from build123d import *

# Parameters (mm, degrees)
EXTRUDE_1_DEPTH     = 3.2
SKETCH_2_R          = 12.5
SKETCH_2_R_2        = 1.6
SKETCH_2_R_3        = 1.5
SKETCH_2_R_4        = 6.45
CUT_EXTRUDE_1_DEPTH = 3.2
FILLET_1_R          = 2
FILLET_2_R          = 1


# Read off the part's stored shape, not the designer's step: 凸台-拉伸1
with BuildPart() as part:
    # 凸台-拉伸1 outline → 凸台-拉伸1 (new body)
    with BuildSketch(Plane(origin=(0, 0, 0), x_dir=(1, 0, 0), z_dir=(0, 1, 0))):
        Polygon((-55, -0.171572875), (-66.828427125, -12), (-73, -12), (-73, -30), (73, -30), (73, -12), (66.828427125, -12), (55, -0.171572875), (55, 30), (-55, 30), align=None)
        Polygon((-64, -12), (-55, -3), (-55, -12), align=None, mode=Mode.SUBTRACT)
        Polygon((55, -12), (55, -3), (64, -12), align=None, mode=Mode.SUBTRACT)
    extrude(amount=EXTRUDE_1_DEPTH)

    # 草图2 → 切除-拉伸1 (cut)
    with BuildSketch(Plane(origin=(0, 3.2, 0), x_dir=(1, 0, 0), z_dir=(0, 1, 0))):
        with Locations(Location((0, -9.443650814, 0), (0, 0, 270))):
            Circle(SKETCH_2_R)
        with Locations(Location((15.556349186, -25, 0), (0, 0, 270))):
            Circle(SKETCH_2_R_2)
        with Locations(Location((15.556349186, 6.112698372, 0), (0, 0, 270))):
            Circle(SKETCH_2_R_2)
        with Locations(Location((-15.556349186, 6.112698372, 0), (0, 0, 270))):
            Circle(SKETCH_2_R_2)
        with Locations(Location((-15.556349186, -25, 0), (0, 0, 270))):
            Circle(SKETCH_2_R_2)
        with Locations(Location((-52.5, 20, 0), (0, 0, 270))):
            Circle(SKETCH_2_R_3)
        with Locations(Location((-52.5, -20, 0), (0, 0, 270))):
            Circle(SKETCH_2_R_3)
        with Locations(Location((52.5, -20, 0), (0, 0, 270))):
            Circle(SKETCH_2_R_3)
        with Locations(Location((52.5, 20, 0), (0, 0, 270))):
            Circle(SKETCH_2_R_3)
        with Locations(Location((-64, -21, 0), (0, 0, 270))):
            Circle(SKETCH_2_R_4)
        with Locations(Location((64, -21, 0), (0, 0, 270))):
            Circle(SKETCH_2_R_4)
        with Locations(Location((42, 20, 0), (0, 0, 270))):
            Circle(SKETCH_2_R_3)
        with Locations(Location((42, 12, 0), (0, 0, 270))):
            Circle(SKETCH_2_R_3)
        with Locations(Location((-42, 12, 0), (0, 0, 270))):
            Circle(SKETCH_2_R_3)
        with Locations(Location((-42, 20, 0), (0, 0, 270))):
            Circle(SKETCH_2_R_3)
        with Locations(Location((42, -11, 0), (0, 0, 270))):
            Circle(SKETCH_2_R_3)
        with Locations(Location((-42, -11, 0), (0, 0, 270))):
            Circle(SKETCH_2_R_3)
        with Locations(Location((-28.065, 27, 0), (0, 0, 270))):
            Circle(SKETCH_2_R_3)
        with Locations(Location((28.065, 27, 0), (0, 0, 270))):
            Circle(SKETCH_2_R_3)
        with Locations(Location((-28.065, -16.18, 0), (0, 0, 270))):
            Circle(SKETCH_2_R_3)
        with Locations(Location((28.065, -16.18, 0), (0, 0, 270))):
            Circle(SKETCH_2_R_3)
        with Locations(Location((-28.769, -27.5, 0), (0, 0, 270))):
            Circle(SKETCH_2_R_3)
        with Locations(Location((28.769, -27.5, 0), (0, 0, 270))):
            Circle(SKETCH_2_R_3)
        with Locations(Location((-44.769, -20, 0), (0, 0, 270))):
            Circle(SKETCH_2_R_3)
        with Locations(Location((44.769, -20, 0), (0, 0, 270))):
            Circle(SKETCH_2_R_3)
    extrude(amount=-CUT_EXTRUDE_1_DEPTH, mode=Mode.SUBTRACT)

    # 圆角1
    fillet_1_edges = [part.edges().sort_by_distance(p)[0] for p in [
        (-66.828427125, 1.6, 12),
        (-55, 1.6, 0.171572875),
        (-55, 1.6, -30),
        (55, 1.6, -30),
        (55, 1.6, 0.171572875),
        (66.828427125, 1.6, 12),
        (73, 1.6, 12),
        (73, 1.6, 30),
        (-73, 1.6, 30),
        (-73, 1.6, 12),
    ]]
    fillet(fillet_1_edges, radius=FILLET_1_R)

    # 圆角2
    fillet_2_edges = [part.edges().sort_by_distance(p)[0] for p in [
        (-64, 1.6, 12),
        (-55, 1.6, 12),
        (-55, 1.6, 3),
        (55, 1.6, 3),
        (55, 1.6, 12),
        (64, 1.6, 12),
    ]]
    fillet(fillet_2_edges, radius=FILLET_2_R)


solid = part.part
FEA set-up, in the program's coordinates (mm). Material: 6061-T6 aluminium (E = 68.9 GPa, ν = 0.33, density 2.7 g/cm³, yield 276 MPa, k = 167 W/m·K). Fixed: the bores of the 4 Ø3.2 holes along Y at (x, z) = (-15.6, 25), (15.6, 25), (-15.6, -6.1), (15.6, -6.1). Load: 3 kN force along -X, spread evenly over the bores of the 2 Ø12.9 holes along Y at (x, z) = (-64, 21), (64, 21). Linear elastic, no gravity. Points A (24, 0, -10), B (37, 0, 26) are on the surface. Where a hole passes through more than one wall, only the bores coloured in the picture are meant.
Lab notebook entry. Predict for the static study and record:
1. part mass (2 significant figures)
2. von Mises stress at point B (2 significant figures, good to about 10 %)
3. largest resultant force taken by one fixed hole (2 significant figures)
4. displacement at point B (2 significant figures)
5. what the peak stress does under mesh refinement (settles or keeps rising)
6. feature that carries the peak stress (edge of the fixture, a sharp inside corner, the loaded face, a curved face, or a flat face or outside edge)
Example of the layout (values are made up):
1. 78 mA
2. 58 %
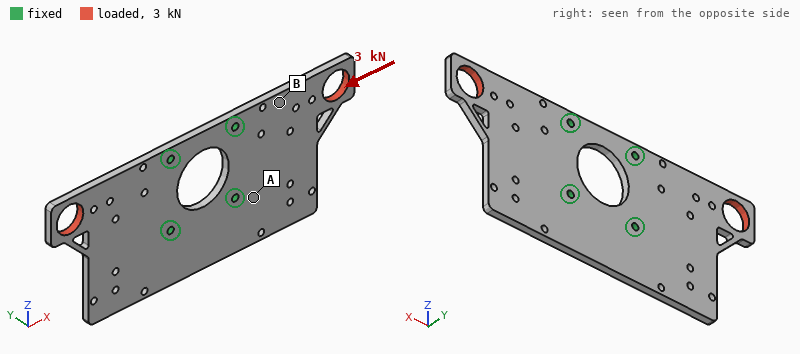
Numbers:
1. 55 g
2. 28 MPa
3. 1.2 kN
4. 12 µm
5. keeps rising
6. a sharp inside corner
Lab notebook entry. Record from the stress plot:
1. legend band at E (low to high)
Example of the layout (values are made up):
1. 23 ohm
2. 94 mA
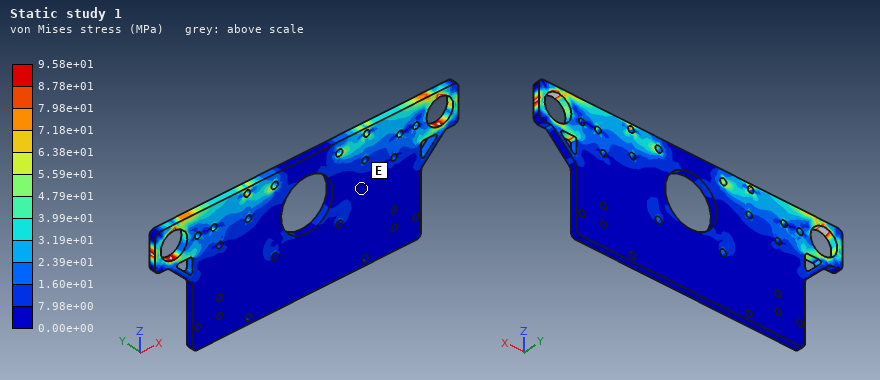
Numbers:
1. 0.00e+00 to 7.98e+00 MPa
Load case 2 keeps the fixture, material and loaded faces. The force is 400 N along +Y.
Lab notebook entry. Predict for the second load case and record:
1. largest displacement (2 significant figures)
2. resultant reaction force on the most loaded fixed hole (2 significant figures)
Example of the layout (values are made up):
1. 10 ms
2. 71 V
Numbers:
1. 1.5 mm
2. 160 N
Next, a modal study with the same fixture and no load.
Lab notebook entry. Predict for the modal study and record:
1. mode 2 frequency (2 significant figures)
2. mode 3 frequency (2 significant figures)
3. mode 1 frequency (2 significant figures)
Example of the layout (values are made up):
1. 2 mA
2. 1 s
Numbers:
1. 1200 Hz
2. 2200 Hz
3. 1200 Hz
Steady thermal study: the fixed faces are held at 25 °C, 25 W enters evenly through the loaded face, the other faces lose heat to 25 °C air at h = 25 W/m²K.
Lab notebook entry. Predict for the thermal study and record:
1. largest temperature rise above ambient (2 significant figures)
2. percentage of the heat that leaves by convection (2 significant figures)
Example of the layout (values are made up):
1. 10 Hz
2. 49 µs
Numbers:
1. 51 K
2. 15 %
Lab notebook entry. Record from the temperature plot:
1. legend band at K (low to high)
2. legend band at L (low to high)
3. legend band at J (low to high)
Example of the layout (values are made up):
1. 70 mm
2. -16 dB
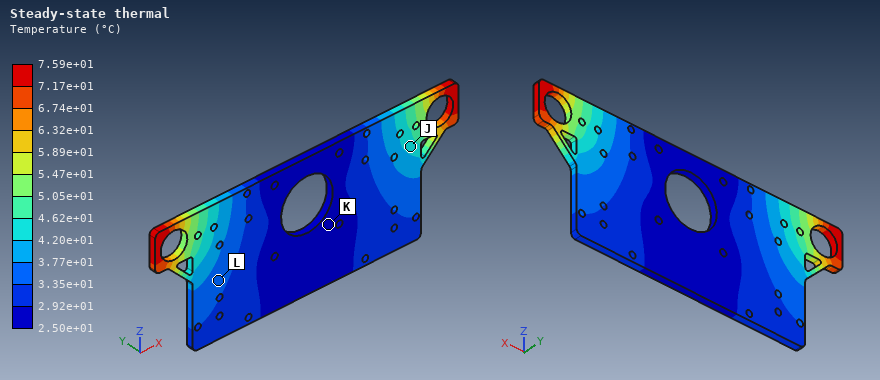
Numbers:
1. 2.50e+01 to 2.92e+01 °C
2. 3.35e+01 to 3.77e+01 °C
3. 4.20e+01 to 4.62e+01 °C
